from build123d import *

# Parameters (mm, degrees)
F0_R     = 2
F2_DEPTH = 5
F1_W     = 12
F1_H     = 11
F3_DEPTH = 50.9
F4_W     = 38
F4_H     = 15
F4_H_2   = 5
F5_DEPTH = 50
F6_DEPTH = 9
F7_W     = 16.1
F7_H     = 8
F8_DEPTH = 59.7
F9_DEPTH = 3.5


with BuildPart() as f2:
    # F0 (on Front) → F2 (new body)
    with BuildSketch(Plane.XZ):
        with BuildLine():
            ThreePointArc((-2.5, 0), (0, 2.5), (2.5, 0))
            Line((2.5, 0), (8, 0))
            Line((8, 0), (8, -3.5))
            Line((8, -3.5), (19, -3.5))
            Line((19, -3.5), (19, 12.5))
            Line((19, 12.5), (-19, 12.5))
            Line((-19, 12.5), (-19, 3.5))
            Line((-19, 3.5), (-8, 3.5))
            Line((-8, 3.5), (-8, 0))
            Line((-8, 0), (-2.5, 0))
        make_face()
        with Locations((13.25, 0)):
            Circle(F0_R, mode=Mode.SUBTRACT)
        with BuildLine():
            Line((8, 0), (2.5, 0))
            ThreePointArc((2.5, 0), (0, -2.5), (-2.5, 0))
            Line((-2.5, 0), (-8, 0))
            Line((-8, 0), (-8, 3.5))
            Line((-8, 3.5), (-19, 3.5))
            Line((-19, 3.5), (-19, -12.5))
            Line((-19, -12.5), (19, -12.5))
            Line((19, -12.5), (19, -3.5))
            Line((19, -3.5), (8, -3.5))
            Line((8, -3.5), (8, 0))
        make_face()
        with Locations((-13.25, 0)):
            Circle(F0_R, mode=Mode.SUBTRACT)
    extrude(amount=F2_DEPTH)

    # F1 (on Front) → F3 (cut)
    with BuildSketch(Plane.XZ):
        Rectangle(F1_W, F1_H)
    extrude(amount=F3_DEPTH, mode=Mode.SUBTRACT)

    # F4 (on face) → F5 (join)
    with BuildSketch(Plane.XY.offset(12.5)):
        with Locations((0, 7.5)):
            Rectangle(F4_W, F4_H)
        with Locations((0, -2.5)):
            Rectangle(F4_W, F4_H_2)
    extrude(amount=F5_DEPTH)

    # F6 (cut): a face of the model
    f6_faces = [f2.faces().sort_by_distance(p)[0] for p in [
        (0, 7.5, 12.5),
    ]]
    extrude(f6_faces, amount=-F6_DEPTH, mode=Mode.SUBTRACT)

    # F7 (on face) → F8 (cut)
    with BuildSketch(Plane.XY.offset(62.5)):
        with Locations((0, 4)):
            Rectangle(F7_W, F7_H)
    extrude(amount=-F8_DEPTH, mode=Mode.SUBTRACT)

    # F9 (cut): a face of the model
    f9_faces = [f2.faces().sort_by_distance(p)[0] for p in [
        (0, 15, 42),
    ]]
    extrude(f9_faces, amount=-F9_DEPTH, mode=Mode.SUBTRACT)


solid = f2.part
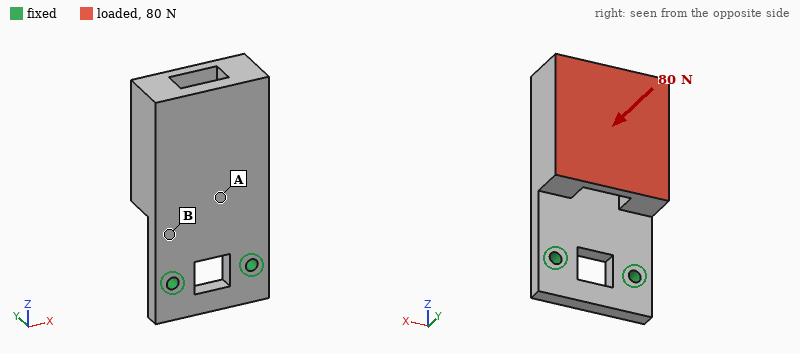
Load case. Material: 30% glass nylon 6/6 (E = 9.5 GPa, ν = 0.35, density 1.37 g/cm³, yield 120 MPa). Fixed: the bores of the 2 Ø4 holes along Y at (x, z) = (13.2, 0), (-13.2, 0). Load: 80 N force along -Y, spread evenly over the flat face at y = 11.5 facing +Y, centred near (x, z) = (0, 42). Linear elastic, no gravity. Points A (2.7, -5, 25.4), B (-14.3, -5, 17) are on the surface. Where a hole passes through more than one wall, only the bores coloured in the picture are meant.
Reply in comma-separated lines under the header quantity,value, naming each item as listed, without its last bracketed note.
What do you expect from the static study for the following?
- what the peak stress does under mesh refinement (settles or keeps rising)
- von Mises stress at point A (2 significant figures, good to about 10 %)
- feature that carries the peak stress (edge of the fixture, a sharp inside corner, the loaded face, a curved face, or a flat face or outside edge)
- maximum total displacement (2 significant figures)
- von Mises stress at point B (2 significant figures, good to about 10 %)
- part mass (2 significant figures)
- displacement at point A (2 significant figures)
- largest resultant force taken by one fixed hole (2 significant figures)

quantity,value
what the peak stress does under mesh refinement,keeps rising
von Mises stress at point A,5.5 MPa
feature that carries the peak stress,edge of the fixture
maximum total displacement,0.99 mm
von Mises stress at point B,13 MPa
part mass,36 g
displacement at point A,0.29 mm
largest resultant force taken by one fixed hole,40 N
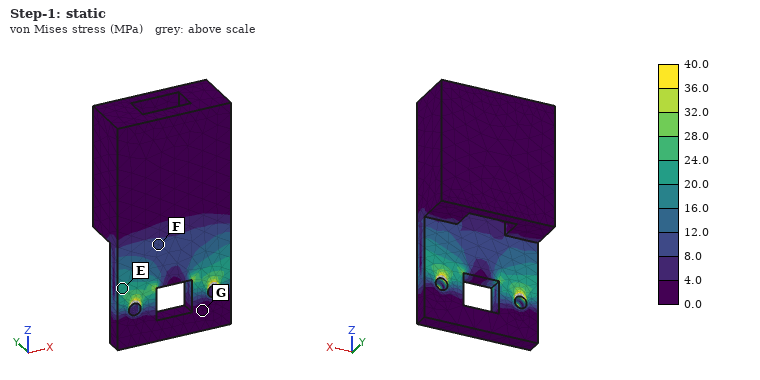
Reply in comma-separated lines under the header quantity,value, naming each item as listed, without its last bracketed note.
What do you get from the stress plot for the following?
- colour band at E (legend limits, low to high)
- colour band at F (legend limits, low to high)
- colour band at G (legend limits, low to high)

quantity,value
colour band at E,20.0 to 24.0 MPa
colour band at F,8.0 to 12.0 MPa
colour band at G,0.0 to 4.0 MPa
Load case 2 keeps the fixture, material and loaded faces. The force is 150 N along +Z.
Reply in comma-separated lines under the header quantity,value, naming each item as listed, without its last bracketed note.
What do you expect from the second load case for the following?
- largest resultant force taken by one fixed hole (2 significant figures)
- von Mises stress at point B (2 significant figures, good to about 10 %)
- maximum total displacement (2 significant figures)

quantity,value
largest resultant force taken by one fixed hole,76 N
von Mises stress at point B,12 MPa
maximum total displacement,0.82 mm
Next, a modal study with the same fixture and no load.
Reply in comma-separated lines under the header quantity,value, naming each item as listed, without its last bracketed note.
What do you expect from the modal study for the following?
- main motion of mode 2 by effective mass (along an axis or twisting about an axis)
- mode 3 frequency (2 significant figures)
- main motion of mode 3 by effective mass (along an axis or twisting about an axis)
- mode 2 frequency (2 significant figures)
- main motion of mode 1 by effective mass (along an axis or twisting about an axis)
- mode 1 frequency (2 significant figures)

quantity,value
main motion of mode 2 by effective mass,along X
mode 3 frequency,2200 Hz
main motion of mode 3 by effective mass,along X
mode 2 frequency,1400 Hz
main motion of mode 1 by effective mass,along Y
mode 1 frequency,320 Hz
